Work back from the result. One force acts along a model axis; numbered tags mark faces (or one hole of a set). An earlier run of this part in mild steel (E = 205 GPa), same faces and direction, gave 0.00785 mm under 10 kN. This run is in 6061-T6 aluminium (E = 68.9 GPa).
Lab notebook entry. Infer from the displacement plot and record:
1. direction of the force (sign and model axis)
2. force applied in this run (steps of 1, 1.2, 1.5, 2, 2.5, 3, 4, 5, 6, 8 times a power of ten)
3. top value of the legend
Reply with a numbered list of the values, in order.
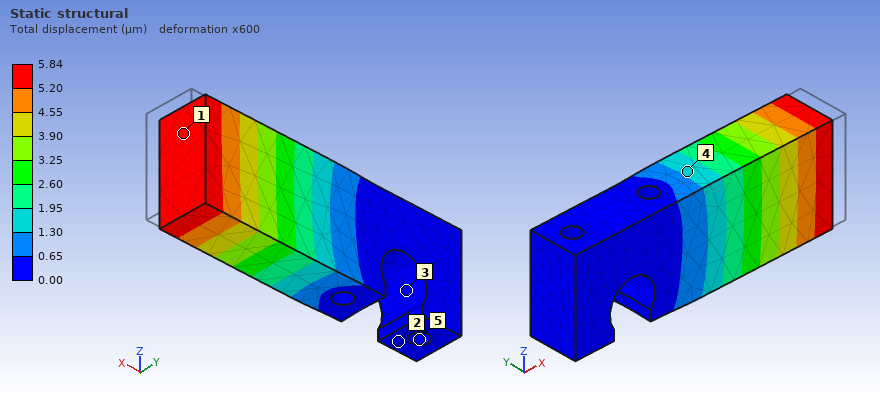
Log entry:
1. -X
2. 2.5 kN
3. 5.84 µm
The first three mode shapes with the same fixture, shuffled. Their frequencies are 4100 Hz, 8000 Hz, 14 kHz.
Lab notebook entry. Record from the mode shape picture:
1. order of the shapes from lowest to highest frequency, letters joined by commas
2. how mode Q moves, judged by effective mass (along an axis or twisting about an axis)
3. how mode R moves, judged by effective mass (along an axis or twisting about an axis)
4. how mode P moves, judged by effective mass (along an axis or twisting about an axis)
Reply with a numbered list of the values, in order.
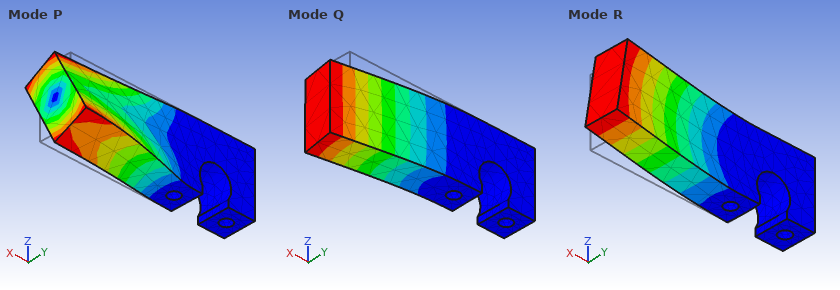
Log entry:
1. Q, R, P
2. along Y
3. along Z
4. twisting about X
